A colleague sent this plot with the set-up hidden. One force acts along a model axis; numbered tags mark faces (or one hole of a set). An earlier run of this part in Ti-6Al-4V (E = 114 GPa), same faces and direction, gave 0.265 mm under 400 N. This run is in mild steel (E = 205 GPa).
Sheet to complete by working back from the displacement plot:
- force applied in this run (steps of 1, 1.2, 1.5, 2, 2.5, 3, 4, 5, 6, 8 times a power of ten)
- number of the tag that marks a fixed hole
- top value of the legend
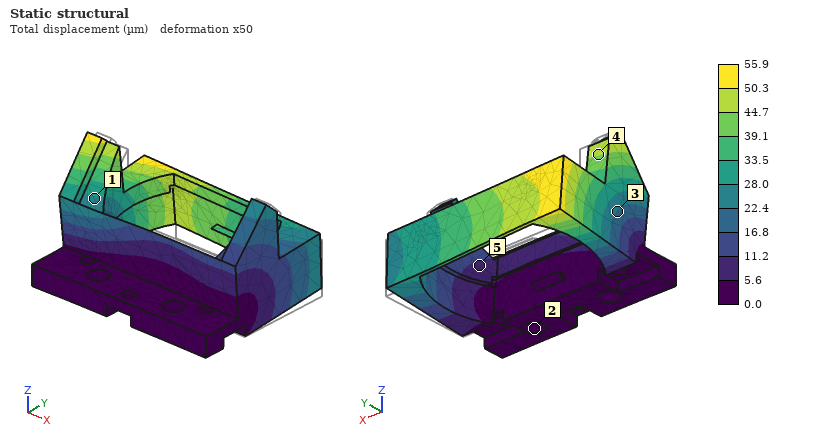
150 N
2
55.9 µm
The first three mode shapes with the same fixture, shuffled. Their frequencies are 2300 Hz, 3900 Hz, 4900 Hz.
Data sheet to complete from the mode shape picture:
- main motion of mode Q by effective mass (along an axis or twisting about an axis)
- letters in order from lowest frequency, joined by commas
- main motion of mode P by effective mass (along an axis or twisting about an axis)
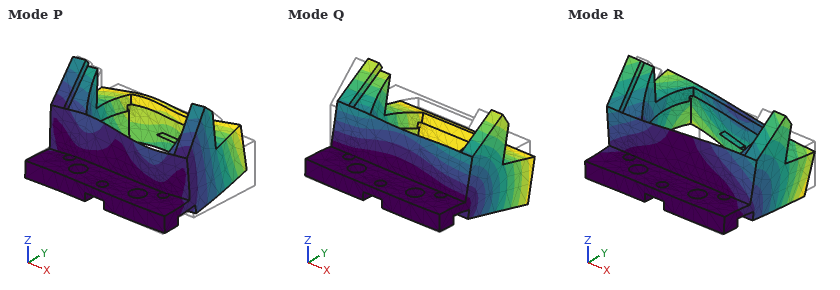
along Z
Q, R, P
along X
